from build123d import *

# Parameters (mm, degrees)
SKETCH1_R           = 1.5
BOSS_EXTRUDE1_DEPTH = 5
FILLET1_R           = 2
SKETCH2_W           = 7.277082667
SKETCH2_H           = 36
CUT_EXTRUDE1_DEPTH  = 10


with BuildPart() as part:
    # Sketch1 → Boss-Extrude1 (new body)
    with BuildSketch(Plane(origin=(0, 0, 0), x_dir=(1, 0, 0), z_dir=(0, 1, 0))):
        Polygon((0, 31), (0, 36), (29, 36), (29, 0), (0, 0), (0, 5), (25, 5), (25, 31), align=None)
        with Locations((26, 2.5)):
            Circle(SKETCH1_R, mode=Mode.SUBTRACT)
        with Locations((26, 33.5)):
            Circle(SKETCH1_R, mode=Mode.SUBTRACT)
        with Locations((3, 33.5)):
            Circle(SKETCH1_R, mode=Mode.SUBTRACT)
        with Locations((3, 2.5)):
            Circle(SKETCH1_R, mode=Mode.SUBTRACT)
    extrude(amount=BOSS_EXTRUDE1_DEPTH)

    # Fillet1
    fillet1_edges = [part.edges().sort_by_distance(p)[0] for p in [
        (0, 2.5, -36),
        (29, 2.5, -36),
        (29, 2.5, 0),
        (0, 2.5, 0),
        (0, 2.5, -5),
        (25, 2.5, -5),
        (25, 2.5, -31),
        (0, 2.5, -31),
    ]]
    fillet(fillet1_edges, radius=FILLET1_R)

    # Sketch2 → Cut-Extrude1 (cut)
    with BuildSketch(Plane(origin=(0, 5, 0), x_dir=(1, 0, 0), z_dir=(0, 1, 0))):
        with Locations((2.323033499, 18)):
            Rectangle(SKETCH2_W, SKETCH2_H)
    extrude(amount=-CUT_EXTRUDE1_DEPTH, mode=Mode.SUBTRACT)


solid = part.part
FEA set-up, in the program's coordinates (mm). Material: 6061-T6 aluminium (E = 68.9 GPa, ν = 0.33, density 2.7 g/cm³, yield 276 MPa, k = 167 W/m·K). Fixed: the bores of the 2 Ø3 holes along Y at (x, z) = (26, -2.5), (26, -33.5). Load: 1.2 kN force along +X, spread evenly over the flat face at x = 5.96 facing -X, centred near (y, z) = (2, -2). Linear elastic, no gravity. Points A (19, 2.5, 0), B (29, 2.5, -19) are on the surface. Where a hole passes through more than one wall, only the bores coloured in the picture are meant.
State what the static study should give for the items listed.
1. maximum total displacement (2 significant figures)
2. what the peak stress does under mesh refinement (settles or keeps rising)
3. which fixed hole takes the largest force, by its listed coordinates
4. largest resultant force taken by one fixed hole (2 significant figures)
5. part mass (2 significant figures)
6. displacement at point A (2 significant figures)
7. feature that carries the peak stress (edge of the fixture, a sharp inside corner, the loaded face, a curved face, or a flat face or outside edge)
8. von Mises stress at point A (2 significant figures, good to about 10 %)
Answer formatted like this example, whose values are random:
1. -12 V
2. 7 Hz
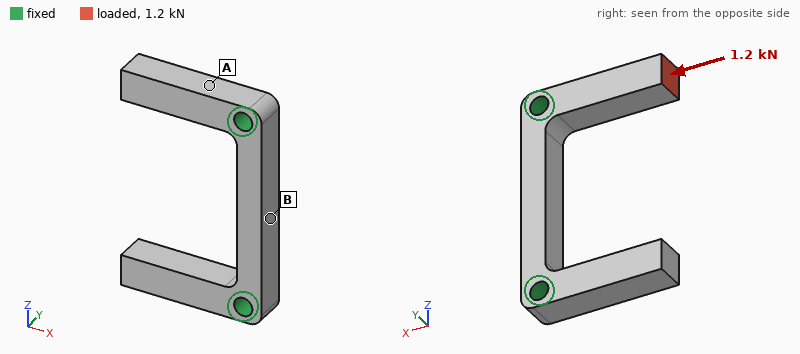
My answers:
1. 14 µm
2. keeps rising
3. (26, -2.5)
4. 1.2 kN
5. 4.3 g
6. 4.5 µm
7. edge of the fixture
8. 48 MPa
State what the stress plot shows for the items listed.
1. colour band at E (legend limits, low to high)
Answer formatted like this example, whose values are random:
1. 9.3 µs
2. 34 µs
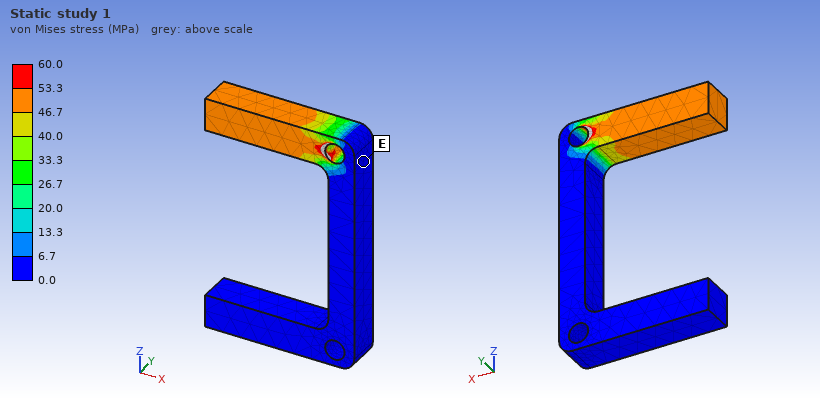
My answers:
1. 0.0 to 6.7 MPa
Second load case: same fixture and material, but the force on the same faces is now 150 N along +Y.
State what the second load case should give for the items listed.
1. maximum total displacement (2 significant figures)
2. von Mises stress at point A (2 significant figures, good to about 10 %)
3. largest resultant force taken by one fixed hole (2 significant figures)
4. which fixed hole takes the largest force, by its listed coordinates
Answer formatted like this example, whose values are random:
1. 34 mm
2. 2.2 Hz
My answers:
1. 0.10 mm
2. 18 MPa
3. 150 N
4. (26, -2.5)
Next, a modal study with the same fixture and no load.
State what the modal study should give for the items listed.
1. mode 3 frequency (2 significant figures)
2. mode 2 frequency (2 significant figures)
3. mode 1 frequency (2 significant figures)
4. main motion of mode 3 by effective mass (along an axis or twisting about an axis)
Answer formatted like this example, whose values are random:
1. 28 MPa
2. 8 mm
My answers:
1. 11 kHz
2. 10 kHz
3. 10 kHz
4. along Y
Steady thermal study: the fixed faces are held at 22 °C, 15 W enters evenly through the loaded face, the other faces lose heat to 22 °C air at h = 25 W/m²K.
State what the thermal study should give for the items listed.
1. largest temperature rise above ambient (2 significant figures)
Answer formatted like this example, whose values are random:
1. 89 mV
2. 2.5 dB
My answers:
1. 67 K
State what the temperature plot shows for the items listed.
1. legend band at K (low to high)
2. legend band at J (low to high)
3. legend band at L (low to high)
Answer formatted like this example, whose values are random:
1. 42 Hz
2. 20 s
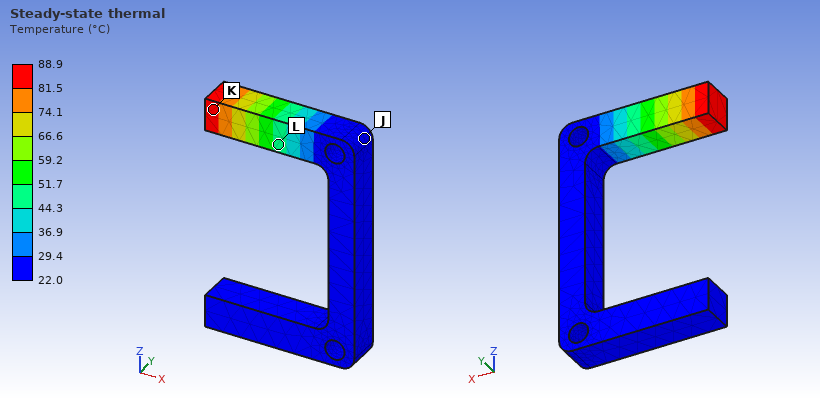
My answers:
1. 81.5 to 88.9 °C
2. 22.0 to 29.4 °C
3. 44.3 to 51.7 °C
